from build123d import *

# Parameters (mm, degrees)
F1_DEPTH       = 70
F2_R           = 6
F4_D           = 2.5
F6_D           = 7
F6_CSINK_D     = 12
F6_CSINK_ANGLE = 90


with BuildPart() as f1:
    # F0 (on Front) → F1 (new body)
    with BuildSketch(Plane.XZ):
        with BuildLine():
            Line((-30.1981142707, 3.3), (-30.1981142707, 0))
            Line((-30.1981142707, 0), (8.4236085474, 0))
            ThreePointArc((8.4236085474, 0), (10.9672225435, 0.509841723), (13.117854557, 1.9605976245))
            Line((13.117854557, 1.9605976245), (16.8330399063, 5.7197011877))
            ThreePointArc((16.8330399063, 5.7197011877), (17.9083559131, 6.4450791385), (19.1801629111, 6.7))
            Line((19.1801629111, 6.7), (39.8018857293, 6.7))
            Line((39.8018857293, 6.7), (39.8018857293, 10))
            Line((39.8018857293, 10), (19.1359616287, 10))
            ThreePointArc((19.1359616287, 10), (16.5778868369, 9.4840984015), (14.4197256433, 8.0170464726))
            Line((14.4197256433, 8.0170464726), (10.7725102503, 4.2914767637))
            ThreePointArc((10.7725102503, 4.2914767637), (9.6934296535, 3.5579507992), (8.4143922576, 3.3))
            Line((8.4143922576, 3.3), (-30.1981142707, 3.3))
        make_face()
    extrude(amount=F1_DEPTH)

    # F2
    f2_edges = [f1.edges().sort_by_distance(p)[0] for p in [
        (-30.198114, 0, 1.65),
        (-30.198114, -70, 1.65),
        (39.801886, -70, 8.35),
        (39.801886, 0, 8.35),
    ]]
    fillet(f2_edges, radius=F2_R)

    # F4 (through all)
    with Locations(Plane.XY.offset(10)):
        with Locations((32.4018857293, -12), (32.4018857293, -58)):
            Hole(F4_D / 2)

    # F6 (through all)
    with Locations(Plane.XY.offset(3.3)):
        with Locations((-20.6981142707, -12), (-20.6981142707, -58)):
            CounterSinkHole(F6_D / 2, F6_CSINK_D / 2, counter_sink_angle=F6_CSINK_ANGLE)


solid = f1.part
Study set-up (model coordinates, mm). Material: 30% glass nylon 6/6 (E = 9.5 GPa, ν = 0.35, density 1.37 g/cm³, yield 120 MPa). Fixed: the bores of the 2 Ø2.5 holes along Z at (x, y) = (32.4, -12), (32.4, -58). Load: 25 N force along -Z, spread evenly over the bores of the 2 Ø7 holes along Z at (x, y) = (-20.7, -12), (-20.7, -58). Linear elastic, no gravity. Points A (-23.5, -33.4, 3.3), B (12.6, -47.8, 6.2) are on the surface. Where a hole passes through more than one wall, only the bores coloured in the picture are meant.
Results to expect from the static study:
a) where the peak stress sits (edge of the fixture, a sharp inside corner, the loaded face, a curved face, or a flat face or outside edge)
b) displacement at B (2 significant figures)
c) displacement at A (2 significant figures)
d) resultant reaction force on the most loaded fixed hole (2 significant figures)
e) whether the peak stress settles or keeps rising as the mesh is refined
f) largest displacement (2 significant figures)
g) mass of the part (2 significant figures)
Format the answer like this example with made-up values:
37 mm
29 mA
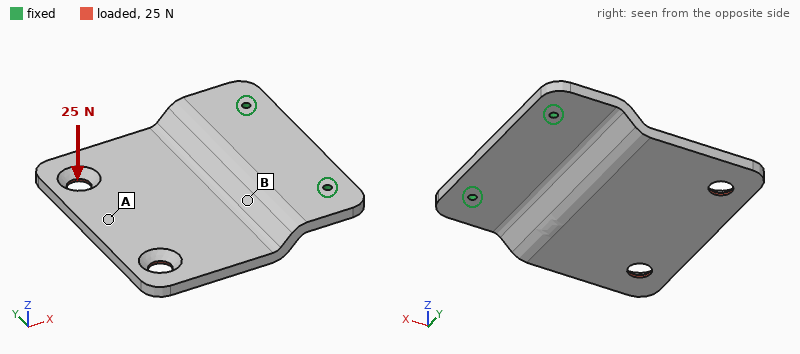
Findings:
edge of the fixture
0.18 mm
0.86 mm
13 N
keeps rising
1.0 mm
22 g
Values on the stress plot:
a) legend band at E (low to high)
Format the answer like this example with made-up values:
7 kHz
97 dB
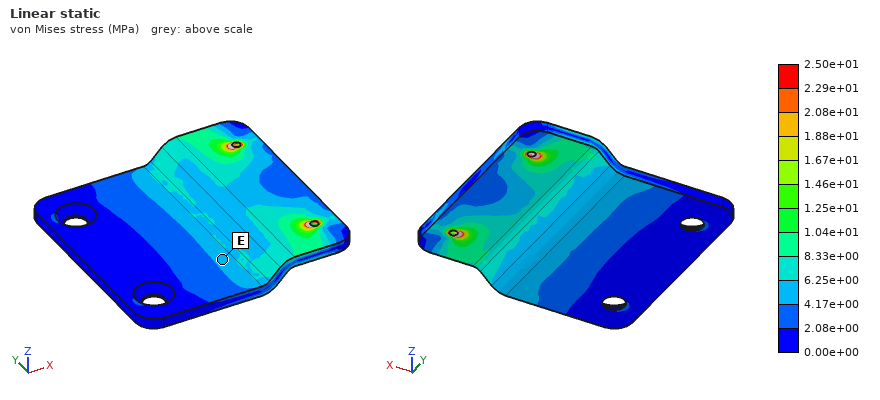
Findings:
4.17e+00 to 6.25e+00 MPa
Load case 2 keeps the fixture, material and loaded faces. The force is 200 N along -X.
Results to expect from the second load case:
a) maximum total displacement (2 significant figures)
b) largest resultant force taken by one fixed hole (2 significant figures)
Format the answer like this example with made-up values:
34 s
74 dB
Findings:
1.2 mm
100 N
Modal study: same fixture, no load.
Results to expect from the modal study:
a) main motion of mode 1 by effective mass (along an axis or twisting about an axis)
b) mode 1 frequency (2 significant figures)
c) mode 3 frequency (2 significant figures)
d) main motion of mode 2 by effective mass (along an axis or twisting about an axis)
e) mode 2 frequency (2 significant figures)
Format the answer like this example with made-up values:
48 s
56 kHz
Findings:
along Z
320 Hz
1900 Hz
twisting about X
800 Hz
